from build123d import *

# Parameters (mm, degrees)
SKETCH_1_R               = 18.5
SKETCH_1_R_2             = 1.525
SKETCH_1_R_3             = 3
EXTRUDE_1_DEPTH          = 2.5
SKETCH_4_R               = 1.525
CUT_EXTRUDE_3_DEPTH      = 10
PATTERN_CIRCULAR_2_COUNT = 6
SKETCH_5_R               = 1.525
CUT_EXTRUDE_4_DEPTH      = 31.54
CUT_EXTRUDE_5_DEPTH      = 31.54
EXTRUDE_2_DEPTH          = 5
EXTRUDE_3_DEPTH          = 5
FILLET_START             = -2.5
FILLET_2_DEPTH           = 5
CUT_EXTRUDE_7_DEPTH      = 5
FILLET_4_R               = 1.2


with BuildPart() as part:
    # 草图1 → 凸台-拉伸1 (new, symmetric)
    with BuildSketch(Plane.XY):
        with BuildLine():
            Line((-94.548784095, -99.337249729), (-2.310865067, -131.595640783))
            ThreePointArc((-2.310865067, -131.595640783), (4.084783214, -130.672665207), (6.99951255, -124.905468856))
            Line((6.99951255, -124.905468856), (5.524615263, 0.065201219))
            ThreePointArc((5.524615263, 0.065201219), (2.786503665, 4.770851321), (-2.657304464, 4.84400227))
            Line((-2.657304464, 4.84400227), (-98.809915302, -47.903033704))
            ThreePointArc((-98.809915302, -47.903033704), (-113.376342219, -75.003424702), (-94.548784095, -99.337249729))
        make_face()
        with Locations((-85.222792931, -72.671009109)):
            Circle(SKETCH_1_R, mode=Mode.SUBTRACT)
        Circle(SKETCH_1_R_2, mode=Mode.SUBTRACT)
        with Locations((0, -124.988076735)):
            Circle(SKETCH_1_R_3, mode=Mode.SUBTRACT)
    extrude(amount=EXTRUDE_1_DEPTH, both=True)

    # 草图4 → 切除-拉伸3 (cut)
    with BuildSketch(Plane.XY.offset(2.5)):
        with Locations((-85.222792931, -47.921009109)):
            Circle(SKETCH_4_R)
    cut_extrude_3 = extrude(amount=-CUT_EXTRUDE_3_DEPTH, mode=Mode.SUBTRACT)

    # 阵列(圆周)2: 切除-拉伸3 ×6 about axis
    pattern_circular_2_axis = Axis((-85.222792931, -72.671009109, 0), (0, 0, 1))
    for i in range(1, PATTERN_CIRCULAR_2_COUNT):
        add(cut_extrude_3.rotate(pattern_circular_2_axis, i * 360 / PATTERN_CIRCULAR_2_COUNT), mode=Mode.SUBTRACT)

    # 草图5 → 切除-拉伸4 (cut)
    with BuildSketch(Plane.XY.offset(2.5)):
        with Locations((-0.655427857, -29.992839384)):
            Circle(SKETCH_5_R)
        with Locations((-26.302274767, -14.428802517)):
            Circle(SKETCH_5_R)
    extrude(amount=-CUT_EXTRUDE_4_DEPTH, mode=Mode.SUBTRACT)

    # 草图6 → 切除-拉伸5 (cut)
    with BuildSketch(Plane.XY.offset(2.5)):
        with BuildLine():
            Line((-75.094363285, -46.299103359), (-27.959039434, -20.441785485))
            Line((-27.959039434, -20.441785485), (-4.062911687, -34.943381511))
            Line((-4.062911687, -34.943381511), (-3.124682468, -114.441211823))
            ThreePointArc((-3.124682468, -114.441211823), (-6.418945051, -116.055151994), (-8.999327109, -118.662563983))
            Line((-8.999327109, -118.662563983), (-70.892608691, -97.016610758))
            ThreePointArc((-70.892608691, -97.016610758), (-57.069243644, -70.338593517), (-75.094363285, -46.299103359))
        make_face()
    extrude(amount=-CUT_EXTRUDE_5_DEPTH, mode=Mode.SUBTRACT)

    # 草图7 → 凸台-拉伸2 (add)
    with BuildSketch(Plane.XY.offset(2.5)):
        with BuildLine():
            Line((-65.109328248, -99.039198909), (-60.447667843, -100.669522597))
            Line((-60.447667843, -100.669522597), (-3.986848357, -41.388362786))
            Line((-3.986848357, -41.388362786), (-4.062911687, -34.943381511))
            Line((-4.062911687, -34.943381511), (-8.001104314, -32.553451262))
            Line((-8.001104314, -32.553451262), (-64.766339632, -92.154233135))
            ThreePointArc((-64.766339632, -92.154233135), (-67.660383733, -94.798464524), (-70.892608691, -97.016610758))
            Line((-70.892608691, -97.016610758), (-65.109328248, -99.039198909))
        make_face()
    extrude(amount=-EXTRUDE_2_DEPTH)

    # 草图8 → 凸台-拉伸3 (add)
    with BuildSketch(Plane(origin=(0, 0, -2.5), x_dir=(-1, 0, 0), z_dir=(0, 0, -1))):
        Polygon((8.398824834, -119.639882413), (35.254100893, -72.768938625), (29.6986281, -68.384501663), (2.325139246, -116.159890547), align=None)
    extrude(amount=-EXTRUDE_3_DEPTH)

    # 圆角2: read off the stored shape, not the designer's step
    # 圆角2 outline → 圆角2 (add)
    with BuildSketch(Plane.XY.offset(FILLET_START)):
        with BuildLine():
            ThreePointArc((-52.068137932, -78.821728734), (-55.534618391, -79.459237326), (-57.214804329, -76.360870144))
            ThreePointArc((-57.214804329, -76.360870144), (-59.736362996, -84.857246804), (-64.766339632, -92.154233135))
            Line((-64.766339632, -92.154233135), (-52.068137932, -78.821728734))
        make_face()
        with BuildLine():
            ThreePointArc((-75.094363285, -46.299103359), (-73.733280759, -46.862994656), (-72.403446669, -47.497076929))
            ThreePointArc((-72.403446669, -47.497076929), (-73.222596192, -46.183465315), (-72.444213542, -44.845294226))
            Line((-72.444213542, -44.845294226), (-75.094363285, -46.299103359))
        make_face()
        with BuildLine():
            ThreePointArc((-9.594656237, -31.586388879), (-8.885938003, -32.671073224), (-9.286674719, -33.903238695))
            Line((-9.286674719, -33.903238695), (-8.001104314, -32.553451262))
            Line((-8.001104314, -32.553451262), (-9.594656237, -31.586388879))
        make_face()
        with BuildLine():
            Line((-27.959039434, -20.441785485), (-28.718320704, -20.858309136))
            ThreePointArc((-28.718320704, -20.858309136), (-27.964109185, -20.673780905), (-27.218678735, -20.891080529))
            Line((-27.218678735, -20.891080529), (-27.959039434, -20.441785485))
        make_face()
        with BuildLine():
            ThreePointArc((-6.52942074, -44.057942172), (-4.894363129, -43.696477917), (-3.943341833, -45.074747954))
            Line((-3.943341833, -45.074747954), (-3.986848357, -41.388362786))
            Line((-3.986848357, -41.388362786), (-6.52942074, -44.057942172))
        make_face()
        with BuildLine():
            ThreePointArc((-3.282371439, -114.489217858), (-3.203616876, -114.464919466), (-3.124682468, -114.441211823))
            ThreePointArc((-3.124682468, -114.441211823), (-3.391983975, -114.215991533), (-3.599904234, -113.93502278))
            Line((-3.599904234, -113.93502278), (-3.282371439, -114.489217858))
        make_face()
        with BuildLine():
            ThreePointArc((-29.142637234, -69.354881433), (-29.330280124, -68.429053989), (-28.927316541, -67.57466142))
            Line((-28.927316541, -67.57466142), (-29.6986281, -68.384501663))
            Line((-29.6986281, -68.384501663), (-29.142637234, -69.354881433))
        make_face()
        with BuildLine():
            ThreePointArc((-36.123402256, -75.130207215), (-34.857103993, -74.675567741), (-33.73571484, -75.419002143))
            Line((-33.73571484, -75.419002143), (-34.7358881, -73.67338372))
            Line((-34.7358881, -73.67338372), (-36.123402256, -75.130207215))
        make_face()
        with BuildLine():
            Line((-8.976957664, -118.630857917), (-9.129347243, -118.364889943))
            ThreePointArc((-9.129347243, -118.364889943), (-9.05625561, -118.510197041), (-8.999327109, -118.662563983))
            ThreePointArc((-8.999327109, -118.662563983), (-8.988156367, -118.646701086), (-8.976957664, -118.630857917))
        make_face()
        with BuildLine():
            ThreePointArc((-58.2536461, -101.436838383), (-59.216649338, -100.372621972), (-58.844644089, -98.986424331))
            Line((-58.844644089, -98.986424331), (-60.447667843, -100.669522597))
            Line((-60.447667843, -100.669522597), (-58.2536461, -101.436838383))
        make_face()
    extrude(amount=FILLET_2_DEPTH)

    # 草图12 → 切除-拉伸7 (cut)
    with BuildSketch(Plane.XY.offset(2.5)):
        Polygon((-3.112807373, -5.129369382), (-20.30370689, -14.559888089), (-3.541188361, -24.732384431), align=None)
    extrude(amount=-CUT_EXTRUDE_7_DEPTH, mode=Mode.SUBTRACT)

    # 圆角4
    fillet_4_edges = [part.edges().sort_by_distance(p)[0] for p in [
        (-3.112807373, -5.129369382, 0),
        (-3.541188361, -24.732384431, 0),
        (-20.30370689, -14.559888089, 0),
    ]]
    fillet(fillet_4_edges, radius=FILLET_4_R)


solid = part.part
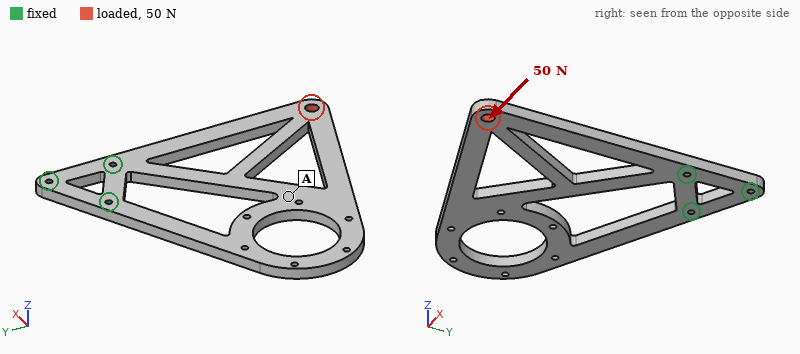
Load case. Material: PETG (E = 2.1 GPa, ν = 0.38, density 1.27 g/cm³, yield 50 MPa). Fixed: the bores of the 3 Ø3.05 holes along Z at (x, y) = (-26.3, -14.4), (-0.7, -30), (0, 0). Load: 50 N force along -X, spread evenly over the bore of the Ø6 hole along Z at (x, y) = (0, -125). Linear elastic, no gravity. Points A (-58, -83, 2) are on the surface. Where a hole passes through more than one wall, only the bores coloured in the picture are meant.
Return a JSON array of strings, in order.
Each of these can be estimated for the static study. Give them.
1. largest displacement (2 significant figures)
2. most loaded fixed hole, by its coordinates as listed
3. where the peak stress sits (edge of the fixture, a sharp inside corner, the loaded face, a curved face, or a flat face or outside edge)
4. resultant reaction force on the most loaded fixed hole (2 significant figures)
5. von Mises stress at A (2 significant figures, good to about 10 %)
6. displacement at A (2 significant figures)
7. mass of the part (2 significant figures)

["2.0 mm", "(-0.7, -30)", "a curved face", "130 N", "2.1 MPa", "1.5 mm", "37 g"]
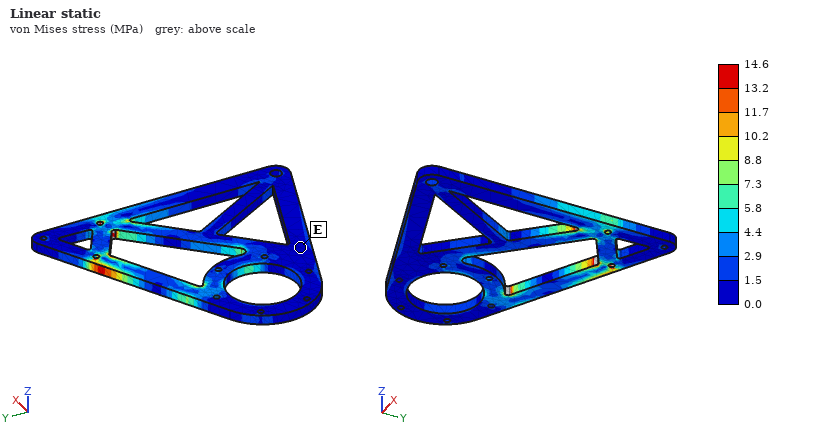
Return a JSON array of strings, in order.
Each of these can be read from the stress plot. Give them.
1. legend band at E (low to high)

["0.0 to 1.5 MPa"]
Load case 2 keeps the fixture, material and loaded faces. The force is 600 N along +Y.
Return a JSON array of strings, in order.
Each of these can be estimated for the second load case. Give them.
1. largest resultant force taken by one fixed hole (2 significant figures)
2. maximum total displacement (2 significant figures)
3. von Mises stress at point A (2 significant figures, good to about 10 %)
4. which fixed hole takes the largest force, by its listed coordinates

["550 N", "0.59 mm", "1.5 MPa", "(-0.7, -30)"]
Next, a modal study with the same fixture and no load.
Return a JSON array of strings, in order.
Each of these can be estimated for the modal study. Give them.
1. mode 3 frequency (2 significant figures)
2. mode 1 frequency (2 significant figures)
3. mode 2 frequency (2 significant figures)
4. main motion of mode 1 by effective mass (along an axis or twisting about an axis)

["190 Hz", "59 Hz", "110 Hz", "along Z"]
